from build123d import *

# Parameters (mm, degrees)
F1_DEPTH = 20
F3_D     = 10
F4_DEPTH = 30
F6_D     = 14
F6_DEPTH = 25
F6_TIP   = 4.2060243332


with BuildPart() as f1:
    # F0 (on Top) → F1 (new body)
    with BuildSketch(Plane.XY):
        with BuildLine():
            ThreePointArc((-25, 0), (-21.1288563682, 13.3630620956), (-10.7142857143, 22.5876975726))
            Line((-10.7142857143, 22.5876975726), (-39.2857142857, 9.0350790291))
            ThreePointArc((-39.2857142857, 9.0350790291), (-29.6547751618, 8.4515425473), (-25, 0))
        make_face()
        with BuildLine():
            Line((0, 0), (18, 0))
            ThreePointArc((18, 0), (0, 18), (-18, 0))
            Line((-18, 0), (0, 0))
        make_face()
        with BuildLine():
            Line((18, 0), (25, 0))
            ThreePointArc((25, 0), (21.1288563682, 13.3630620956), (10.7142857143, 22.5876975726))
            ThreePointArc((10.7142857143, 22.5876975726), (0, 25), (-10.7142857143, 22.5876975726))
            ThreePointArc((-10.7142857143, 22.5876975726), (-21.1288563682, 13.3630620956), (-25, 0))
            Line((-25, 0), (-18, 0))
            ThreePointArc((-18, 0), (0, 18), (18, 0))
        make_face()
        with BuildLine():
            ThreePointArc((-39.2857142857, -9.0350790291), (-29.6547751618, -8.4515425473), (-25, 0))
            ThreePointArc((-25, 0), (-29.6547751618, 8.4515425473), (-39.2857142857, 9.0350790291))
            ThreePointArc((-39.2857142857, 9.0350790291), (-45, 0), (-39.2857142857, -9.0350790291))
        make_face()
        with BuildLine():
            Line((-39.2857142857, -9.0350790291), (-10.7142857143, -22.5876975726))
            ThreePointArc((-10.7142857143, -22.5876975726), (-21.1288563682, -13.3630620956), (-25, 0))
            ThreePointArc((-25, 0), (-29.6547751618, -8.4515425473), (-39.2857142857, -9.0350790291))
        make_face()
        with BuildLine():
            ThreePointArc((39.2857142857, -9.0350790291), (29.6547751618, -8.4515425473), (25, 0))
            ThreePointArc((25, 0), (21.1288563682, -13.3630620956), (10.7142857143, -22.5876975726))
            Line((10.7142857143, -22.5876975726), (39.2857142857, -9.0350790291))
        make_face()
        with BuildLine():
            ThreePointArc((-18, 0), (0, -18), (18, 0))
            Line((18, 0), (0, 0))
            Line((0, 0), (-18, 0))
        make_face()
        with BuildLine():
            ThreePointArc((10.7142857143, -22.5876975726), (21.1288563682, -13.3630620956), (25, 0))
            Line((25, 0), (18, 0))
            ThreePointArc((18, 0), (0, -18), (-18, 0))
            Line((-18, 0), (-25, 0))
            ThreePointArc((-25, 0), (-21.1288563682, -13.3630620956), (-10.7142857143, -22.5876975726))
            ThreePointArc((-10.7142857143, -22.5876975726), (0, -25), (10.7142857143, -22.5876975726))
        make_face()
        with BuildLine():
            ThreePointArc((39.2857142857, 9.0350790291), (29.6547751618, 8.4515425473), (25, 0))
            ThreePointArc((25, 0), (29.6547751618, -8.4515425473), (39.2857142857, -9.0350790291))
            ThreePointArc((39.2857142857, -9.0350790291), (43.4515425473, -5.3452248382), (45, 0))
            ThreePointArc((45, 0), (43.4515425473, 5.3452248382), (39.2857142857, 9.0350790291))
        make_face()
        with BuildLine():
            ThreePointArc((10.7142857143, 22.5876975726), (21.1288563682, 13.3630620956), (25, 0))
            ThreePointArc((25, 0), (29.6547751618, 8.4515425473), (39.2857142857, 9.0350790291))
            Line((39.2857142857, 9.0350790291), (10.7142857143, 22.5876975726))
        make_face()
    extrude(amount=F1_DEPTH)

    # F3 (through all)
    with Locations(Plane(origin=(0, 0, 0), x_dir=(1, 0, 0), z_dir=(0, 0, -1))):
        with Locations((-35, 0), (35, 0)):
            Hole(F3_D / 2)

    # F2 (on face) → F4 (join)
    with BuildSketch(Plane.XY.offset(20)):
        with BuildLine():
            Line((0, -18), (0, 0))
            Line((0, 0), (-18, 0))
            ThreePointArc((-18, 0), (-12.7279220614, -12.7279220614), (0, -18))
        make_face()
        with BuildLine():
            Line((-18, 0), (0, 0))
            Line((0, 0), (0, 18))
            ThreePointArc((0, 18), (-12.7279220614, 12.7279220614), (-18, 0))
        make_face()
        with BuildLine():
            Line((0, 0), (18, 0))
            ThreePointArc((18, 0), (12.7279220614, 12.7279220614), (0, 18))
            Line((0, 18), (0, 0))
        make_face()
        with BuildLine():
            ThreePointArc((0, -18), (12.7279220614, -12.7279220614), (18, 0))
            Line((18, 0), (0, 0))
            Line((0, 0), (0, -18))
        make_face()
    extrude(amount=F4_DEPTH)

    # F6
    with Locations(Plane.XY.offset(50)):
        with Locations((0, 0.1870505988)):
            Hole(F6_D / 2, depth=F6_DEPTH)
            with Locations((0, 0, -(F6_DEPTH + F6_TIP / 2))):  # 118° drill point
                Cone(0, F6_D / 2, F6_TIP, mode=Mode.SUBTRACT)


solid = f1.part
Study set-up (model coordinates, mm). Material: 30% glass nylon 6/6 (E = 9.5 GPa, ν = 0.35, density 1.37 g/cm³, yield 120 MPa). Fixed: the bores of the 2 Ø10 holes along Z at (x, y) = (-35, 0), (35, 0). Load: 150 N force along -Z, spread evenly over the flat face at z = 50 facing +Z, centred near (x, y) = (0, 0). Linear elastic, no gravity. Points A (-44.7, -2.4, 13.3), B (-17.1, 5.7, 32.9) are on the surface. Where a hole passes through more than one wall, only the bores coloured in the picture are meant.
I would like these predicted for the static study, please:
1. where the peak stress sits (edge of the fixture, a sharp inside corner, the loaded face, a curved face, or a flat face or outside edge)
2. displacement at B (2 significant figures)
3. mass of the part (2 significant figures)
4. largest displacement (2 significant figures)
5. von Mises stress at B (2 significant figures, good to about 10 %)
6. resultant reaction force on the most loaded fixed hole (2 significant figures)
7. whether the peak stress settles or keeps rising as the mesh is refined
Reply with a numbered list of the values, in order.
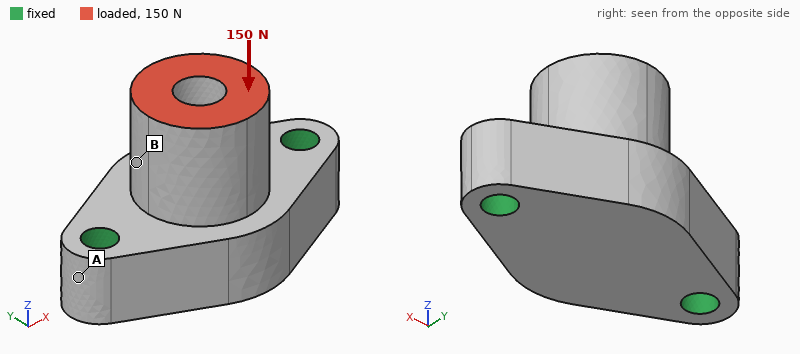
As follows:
1. edge of the fixture
2. 1.6 µm
3. 110 g
4. 1.9 µm
5. 0.19 MPa
6. 77 N
7. keeps rising
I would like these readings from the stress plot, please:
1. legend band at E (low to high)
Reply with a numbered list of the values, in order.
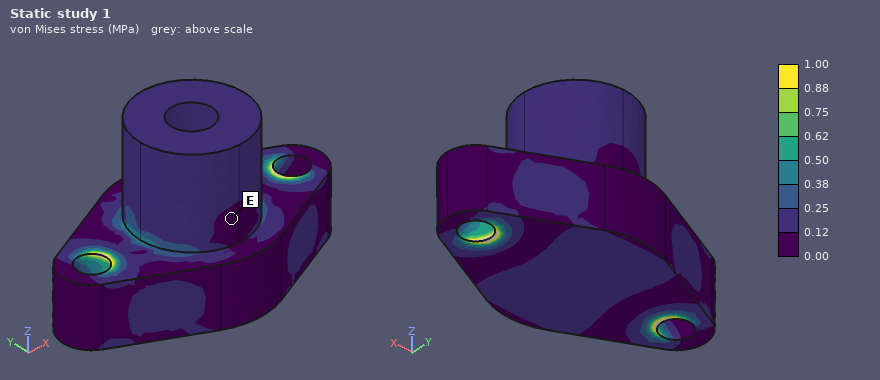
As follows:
1. 0.00 to 0.12 MPa
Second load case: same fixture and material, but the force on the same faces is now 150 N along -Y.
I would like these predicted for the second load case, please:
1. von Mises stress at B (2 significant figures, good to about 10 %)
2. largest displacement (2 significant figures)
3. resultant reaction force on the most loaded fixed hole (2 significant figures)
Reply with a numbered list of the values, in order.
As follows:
1. 0.42 MPa
2. 21 µm
3. 75 N
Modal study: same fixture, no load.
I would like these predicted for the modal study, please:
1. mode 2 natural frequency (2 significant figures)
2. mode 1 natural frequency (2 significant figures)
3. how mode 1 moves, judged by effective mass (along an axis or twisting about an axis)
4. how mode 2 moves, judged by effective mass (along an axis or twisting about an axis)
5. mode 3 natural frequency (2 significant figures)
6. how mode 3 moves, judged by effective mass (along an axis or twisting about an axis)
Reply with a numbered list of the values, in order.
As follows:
1. 5600 Hz
2. 3100 Hz
3. along Y
4. along Z
5. 6000 Hz
6. along X
